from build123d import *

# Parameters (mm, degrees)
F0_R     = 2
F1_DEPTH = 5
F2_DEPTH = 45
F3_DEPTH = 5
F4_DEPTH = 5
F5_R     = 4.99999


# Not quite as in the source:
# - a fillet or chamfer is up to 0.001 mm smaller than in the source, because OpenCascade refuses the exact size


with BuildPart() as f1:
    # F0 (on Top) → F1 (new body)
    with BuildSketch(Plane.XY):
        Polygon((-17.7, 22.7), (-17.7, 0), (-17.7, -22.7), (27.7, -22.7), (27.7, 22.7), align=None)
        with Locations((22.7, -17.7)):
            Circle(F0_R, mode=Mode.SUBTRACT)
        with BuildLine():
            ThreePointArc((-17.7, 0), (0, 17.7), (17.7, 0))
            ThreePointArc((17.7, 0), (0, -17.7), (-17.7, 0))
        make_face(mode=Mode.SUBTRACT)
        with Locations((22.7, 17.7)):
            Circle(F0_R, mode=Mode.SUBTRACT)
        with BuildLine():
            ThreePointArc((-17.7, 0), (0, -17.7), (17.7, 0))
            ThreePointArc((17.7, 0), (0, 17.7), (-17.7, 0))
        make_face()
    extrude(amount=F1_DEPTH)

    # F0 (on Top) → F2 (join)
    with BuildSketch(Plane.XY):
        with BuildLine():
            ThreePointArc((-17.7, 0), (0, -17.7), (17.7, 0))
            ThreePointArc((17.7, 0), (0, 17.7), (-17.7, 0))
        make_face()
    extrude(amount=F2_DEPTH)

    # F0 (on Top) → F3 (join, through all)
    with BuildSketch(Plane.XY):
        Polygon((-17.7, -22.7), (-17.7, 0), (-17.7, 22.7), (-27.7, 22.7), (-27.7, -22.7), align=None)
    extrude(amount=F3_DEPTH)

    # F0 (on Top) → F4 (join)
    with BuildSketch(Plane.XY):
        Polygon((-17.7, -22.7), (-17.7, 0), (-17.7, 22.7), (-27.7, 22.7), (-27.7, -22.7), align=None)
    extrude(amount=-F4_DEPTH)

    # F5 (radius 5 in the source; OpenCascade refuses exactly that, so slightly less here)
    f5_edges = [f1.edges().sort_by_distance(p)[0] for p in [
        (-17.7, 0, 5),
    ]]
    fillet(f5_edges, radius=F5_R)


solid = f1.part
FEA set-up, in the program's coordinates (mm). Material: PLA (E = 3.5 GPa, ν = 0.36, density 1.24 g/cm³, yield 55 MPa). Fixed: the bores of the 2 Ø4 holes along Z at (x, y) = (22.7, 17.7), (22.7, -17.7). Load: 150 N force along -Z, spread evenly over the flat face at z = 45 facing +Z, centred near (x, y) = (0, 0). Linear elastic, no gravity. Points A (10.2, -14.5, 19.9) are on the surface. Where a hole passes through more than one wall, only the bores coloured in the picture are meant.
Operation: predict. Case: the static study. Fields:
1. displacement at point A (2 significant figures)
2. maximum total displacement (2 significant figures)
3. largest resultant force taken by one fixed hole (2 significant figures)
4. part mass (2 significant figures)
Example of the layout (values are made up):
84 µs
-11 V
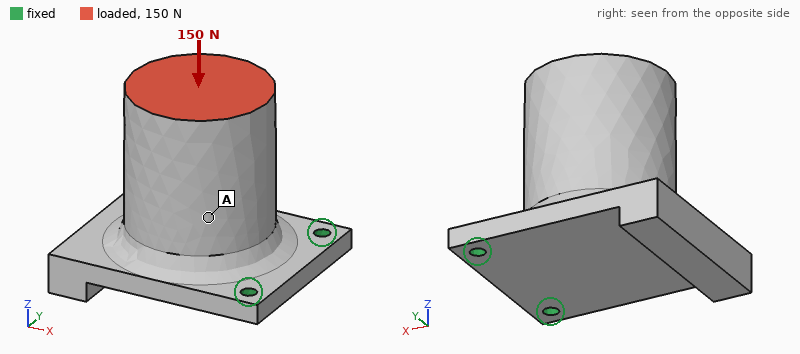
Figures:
0.35 mm
1.00 mm
75 N
68 g
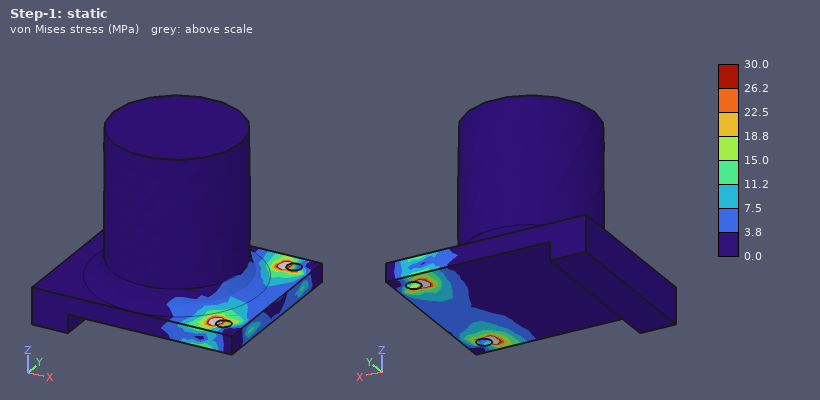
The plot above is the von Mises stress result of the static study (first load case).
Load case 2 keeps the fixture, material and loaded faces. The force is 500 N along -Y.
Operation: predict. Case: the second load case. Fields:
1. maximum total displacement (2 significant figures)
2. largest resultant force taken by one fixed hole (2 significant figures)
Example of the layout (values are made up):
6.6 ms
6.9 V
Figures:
0.77 mm
760 N
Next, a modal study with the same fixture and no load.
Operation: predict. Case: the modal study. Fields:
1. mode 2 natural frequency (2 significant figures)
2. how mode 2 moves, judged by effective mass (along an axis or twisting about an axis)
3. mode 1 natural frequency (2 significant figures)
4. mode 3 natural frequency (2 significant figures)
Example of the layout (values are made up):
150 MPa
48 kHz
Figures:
930 Hz
along Y
240 Hz
2000 Hz
